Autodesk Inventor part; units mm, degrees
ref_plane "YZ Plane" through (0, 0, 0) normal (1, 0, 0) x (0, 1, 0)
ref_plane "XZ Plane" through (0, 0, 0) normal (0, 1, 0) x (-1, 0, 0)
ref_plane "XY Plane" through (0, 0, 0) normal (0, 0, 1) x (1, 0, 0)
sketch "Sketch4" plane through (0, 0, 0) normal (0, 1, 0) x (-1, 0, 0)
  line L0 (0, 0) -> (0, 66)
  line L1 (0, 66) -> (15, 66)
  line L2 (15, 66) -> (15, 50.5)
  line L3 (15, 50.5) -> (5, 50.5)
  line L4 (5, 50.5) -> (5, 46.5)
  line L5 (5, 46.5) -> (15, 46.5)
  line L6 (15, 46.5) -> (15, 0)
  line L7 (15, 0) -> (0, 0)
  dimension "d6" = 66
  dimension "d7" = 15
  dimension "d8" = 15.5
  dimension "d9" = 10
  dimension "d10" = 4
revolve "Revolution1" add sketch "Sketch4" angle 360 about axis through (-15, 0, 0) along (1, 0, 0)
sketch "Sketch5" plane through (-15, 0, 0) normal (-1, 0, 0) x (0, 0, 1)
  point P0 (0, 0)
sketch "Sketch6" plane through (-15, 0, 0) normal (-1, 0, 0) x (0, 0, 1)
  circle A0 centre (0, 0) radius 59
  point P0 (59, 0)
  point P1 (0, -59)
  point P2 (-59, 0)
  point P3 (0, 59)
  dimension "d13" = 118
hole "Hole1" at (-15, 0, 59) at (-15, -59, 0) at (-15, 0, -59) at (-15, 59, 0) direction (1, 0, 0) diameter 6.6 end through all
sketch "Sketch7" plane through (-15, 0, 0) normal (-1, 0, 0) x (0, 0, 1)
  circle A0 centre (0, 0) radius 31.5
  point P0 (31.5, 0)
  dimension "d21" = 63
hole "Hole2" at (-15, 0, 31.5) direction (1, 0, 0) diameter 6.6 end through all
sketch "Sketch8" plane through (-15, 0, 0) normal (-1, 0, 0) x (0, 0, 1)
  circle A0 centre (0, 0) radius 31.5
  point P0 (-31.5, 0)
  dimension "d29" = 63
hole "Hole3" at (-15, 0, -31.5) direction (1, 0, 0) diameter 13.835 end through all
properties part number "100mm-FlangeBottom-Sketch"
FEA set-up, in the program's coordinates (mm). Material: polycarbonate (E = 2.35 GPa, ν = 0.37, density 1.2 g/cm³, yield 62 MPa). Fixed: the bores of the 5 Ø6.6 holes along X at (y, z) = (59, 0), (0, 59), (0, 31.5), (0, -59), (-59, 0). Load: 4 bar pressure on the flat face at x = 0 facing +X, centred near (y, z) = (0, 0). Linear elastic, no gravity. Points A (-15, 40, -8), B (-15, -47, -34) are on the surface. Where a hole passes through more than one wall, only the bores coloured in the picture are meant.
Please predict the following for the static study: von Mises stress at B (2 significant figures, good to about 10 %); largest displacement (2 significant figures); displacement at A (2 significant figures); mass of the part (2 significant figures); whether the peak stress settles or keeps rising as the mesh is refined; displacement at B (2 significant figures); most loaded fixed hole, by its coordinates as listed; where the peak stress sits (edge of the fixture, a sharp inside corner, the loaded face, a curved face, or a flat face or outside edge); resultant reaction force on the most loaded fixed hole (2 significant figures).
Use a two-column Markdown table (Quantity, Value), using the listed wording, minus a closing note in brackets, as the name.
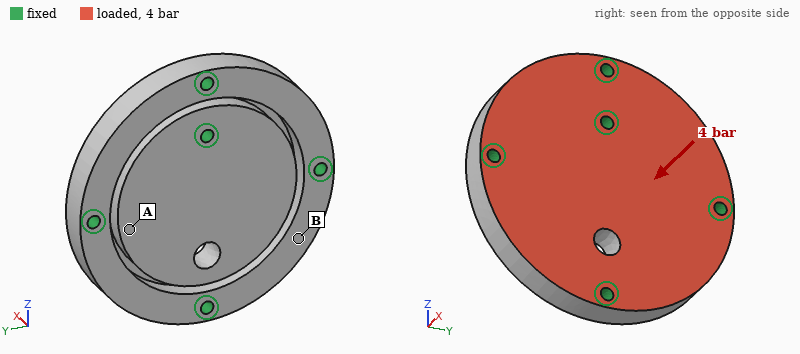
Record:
| Quantity | Value |
|---|---|
| von Mises stress at B | 4.4 MPa |
| largest displacement | 0.20 mm |
| displacement at A | 0.13 mm |
| mass of the part | 230 g |
| whether the peak stress settles or keeps rising as the mesh is refined | keeps rising |
| displacement at B | 0.17 mm |
| most loaded fixed hole, by its coordinates as listed | (0, 31.5) |
| where the peak stress sits | edge of the fixture |
| resultant reaction force on the most loaded fixed hole | 1.5 kN |
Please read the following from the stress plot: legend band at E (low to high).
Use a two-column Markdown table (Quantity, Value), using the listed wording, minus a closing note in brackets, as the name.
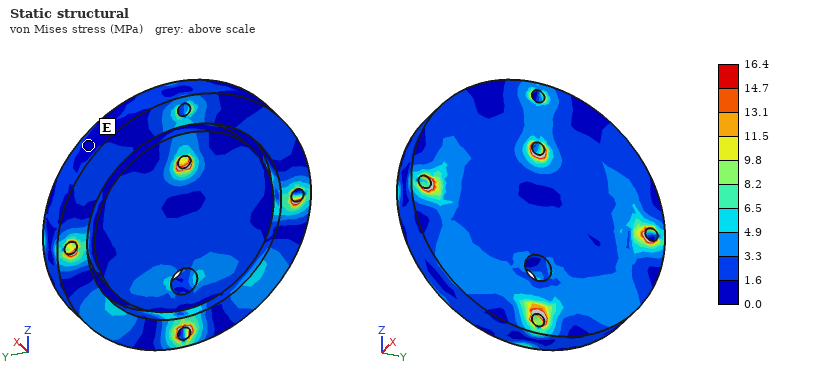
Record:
| Quantity | Value |
|---|---|
| legend band at E | 0.0 to 1.6 MPa |
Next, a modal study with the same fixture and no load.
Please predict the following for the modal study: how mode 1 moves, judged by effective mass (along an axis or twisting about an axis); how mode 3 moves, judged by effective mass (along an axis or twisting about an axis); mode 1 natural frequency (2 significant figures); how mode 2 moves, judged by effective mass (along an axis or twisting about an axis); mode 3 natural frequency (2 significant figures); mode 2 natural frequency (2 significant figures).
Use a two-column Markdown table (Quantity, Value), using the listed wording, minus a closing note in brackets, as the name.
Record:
| Quantity | Value |
|---|---|
| how mode 1 moves, judged by effective mass | along X |
| how mode 3 moves, judged by effective mass | twisting about Z |
| mode 1 natural frequency | 1900 Hz |
| how mode 2 moves, judged by effective mass | twisting about Z |
| mode 3 natural frequency | 2300 Hz |
| mode 2 natural frequency | 2100 Hz |
